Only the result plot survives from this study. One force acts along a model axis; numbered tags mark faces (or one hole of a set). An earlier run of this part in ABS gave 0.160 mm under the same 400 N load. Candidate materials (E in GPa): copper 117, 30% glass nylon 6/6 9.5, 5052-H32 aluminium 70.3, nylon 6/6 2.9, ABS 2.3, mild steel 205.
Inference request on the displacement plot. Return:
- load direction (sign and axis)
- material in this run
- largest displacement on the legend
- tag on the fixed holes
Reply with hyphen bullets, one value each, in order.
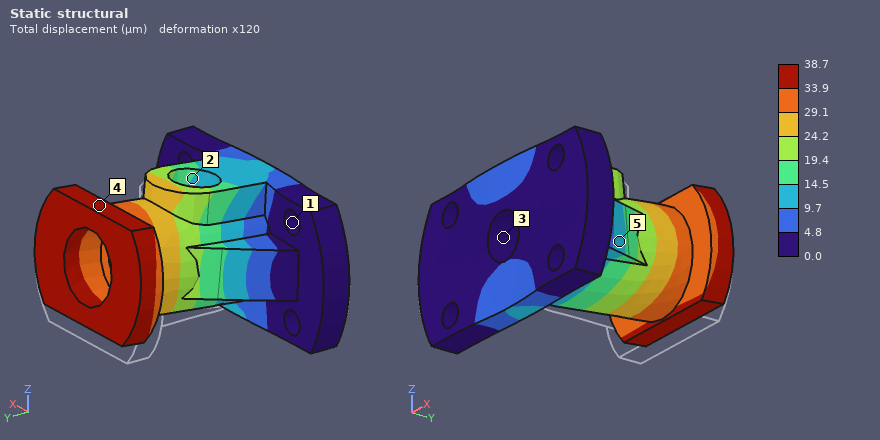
- +Z
- 30% glass nylon 6/6
- 38.7 µm
- 1
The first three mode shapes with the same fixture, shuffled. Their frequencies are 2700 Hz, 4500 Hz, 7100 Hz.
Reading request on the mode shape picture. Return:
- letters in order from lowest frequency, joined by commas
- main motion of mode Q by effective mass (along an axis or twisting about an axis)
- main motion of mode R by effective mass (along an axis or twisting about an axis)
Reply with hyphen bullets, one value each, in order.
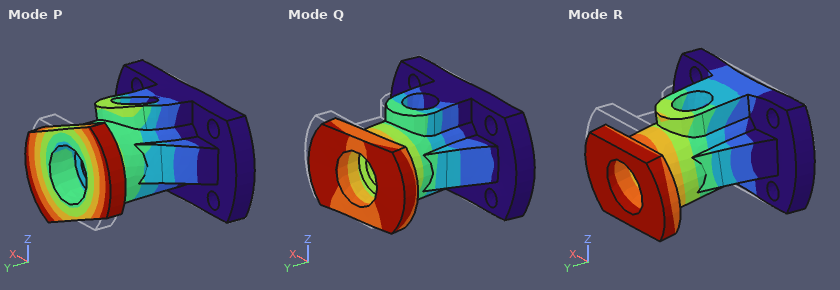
- R, Q, P
- along X
- along Z
